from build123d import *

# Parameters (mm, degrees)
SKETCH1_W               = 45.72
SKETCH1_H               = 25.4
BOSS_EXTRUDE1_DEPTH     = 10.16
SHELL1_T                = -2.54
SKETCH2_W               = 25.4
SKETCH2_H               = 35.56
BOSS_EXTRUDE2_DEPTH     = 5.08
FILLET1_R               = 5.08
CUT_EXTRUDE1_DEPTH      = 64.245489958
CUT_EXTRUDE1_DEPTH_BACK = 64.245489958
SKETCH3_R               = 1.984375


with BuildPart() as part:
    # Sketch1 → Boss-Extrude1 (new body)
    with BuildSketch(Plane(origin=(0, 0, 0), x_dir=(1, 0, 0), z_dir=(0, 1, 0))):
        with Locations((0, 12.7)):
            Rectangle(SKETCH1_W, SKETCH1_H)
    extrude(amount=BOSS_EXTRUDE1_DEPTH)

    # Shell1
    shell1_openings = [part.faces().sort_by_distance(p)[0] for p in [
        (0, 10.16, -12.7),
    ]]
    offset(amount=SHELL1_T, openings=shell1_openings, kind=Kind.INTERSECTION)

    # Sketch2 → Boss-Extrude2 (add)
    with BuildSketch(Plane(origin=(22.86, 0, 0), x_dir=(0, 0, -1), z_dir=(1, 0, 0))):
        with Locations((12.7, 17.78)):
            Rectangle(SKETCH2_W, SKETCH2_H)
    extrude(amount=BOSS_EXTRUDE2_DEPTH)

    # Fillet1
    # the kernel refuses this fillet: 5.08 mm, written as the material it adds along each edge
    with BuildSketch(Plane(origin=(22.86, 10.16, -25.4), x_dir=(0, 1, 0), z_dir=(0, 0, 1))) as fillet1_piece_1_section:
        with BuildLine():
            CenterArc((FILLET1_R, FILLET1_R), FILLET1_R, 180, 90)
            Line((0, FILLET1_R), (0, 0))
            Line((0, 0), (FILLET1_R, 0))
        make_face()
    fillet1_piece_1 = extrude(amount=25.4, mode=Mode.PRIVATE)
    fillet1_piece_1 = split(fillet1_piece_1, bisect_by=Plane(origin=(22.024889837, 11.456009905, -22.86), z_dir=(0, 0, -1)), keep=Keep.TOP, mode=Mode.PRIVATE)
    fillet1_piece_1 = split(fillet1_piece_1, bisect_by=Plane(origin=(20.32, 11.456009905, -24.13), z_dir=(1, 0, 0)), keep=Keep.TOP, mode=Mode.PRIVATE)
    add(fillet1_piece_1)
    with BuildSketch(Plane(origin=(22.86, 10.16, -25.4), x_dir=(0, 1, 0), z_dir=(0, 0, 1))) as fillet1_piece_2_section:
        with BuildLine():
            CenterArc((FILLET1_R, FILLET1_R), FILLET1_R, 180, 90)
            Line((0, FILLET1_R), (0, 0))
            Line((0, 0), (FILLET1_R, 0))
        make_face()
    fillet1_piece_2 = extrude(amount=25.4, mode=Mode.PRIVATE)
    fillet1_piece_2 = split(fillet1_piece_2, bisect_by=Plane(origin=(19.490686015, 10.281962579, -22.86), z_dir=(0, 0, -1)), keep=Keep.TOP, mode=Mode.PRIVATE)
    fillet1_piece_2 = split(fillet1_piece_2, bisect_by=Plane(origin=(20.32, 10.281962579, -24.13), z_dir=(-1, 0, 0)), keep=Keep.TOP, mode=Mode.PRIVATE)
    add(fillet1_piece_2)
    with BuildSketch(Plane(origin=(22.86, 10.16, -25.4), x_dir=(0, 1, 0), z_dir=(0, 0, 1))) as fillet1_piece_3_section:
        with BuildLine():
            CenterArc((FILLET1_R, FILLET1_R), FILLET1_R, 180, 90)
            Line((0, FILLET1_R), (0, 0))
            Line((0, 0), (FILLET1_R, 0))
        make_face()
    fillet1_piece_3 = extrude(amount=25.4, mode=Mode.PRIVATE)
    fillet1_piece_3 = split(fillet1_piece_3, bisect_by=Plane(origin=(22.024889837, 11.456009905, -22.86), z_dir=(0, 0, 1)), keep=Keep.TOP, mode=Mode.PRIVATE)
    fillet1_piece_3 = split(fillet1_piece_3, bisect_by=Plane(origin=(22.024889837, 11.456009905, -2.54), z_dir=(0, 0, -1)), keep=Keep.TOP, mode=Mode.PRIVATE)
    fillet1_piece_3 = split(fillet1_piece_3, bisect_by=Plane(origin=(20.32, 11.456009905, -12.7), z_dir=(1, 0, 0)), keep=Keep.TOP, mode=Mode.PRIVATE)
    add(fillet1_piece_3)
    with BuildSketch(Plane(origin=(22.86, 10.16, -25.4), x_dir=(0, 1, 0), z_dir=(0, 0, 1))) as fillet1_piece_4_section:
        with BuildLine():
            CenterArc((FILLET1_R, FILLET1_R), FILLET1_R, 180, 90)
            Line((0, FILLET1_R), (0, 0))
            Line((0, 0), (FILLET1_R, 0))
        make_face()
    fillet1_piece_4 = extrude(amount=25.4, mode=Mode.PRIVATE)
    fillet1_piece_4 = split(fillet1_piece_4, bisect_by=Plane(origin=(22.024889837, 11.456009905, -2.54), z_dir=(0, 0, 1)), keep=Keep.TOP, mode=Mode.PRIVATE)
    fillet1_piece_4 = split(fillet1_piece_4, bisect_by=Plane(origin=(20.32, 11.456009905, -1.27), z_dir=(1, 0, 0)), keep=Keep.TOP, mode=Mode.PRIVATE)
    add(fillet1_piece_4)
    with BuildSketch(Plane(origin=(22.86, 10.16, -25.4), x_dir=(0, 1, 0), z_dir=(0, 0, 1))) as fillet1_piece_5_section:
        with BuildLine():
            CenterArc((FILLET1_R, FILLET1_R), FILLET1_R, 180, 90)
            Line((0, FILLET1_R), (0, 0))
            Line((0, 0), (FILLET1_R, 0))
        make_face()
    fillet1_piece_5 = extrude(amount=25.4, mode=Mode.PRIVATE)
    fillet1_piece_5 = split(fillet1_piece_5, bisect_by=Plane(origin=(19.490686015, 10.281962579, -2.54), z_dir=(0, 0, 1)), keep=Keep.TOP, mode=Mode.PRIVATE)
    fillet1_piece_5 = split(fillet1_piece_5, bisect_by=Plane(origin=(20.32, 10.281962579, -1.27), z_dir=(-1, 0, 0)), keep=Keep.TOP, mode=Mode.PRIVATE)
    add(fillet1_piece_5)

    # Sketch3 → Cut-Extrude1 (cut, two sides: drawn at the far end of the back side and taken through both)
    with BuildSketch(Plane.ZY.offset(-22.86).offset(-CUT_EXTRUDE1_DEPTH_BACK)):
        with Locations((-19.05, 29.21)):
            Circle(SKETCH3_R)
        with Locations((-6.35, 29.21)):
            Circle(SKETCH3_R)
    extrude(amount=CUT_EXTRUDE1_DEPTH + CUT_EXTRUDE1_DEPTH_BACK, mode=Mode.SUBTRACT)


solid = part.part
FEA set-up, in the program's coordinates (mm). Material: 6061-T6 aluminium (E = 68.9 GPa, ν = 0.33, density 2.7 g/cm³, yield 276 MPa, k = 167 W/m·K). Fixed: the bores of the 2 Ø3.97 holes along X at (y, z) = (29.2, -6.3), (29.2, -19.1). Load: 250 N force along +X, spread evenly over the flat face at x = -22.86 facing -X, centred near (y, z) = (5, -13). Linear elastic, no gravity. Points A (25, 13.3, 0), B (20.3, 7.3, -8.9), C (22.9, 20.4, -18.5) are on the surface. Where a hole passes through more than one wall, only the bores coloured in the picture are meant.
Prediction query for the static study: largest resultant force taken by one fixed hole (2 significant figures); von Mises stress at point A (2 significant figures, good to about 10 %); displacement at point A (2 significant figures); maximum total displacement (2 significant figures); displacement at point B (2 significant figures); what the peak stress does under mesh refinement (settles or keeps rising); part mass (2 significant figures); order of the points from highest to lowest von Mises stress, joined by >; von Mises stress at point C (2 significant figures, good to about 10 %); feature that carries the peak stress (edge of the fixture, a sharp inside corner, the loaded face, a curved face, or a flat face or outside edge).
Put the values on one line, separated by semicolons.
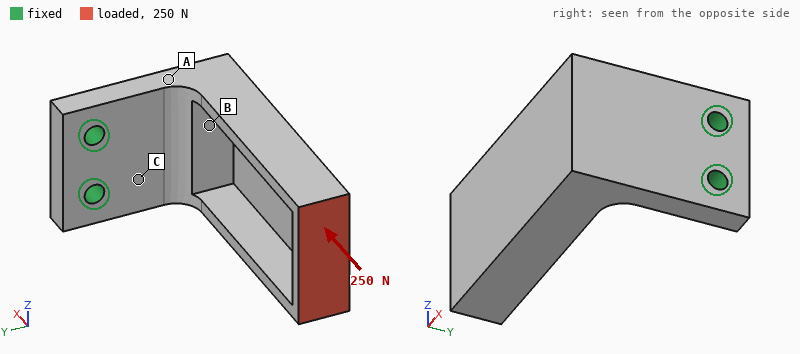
130 N; 13 MPa; 0.028 mm; 0.17 mm; 0.051 mm; keeps rising; 27 g; C > A > B; 32 MPa; edge of the fixture
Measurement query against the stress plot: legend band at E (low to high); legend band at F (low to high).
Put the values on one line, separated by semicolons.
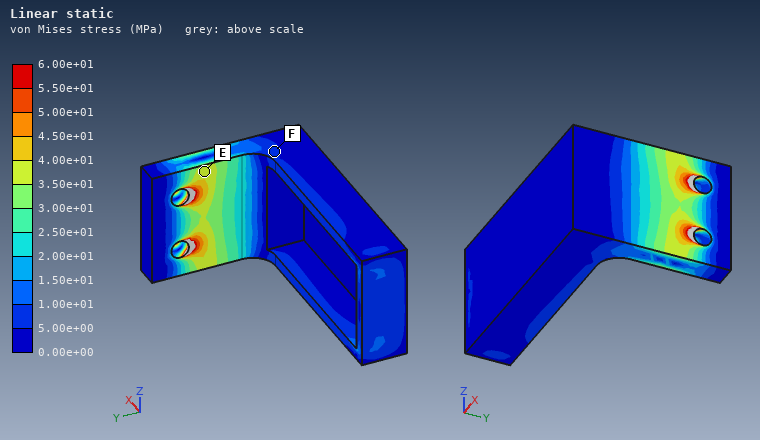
3.50e+01 to 4.00e+01 MPa; 5.00e+00 to 1.00e+01 MPa
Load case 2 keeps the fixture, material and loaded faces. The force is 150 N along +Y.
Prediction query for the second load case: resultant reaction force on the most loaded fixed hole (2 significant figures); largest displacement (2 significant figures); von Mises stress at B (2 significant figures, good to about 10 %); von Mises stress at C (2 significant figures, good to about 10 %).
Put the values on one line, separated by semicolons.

78 N; 0.45 mm; 24 MPa; 64 MPa
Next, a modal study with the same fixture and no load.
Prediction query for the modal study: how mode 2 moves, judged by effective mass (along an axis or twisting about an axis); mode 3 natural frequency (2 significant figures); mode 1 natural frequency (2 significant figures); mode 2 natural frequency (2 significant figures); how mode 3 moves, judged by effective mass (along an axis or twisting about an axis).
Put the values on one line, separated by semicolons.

along Z; 4500 Hz; 1200 Hz; 1800 Hz; along X
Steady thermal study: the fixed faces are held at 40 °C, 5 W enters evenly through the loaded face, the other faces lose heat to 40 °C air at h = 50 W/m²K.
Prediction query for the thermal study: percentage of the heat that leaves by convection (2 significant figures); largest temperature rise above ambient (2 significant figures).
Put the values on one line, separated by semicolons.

37 %; 14 K
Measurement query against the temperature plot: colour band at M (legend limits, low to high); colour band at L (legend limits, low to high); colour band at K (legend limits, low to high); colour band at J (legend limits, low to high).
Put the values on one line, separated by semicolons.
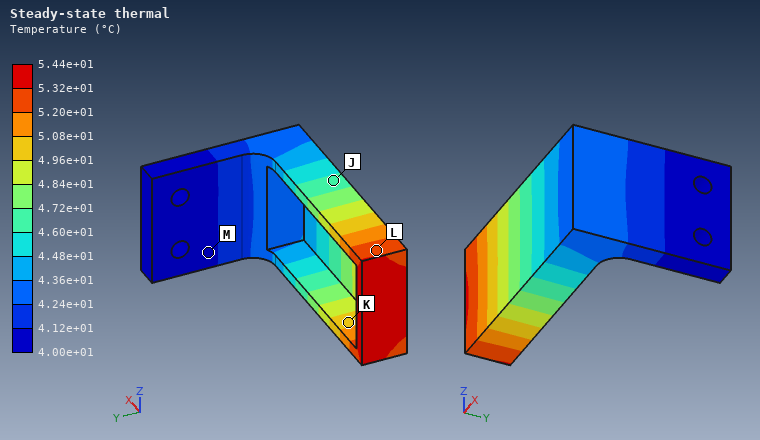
4.00e+01 to 4.12e+01 °C; 5.20e+01 to 5.32e+01 °C; 4.96e+01 to 5.08e+01 °C; 4.60e+01 to 4.72e+01 °C
